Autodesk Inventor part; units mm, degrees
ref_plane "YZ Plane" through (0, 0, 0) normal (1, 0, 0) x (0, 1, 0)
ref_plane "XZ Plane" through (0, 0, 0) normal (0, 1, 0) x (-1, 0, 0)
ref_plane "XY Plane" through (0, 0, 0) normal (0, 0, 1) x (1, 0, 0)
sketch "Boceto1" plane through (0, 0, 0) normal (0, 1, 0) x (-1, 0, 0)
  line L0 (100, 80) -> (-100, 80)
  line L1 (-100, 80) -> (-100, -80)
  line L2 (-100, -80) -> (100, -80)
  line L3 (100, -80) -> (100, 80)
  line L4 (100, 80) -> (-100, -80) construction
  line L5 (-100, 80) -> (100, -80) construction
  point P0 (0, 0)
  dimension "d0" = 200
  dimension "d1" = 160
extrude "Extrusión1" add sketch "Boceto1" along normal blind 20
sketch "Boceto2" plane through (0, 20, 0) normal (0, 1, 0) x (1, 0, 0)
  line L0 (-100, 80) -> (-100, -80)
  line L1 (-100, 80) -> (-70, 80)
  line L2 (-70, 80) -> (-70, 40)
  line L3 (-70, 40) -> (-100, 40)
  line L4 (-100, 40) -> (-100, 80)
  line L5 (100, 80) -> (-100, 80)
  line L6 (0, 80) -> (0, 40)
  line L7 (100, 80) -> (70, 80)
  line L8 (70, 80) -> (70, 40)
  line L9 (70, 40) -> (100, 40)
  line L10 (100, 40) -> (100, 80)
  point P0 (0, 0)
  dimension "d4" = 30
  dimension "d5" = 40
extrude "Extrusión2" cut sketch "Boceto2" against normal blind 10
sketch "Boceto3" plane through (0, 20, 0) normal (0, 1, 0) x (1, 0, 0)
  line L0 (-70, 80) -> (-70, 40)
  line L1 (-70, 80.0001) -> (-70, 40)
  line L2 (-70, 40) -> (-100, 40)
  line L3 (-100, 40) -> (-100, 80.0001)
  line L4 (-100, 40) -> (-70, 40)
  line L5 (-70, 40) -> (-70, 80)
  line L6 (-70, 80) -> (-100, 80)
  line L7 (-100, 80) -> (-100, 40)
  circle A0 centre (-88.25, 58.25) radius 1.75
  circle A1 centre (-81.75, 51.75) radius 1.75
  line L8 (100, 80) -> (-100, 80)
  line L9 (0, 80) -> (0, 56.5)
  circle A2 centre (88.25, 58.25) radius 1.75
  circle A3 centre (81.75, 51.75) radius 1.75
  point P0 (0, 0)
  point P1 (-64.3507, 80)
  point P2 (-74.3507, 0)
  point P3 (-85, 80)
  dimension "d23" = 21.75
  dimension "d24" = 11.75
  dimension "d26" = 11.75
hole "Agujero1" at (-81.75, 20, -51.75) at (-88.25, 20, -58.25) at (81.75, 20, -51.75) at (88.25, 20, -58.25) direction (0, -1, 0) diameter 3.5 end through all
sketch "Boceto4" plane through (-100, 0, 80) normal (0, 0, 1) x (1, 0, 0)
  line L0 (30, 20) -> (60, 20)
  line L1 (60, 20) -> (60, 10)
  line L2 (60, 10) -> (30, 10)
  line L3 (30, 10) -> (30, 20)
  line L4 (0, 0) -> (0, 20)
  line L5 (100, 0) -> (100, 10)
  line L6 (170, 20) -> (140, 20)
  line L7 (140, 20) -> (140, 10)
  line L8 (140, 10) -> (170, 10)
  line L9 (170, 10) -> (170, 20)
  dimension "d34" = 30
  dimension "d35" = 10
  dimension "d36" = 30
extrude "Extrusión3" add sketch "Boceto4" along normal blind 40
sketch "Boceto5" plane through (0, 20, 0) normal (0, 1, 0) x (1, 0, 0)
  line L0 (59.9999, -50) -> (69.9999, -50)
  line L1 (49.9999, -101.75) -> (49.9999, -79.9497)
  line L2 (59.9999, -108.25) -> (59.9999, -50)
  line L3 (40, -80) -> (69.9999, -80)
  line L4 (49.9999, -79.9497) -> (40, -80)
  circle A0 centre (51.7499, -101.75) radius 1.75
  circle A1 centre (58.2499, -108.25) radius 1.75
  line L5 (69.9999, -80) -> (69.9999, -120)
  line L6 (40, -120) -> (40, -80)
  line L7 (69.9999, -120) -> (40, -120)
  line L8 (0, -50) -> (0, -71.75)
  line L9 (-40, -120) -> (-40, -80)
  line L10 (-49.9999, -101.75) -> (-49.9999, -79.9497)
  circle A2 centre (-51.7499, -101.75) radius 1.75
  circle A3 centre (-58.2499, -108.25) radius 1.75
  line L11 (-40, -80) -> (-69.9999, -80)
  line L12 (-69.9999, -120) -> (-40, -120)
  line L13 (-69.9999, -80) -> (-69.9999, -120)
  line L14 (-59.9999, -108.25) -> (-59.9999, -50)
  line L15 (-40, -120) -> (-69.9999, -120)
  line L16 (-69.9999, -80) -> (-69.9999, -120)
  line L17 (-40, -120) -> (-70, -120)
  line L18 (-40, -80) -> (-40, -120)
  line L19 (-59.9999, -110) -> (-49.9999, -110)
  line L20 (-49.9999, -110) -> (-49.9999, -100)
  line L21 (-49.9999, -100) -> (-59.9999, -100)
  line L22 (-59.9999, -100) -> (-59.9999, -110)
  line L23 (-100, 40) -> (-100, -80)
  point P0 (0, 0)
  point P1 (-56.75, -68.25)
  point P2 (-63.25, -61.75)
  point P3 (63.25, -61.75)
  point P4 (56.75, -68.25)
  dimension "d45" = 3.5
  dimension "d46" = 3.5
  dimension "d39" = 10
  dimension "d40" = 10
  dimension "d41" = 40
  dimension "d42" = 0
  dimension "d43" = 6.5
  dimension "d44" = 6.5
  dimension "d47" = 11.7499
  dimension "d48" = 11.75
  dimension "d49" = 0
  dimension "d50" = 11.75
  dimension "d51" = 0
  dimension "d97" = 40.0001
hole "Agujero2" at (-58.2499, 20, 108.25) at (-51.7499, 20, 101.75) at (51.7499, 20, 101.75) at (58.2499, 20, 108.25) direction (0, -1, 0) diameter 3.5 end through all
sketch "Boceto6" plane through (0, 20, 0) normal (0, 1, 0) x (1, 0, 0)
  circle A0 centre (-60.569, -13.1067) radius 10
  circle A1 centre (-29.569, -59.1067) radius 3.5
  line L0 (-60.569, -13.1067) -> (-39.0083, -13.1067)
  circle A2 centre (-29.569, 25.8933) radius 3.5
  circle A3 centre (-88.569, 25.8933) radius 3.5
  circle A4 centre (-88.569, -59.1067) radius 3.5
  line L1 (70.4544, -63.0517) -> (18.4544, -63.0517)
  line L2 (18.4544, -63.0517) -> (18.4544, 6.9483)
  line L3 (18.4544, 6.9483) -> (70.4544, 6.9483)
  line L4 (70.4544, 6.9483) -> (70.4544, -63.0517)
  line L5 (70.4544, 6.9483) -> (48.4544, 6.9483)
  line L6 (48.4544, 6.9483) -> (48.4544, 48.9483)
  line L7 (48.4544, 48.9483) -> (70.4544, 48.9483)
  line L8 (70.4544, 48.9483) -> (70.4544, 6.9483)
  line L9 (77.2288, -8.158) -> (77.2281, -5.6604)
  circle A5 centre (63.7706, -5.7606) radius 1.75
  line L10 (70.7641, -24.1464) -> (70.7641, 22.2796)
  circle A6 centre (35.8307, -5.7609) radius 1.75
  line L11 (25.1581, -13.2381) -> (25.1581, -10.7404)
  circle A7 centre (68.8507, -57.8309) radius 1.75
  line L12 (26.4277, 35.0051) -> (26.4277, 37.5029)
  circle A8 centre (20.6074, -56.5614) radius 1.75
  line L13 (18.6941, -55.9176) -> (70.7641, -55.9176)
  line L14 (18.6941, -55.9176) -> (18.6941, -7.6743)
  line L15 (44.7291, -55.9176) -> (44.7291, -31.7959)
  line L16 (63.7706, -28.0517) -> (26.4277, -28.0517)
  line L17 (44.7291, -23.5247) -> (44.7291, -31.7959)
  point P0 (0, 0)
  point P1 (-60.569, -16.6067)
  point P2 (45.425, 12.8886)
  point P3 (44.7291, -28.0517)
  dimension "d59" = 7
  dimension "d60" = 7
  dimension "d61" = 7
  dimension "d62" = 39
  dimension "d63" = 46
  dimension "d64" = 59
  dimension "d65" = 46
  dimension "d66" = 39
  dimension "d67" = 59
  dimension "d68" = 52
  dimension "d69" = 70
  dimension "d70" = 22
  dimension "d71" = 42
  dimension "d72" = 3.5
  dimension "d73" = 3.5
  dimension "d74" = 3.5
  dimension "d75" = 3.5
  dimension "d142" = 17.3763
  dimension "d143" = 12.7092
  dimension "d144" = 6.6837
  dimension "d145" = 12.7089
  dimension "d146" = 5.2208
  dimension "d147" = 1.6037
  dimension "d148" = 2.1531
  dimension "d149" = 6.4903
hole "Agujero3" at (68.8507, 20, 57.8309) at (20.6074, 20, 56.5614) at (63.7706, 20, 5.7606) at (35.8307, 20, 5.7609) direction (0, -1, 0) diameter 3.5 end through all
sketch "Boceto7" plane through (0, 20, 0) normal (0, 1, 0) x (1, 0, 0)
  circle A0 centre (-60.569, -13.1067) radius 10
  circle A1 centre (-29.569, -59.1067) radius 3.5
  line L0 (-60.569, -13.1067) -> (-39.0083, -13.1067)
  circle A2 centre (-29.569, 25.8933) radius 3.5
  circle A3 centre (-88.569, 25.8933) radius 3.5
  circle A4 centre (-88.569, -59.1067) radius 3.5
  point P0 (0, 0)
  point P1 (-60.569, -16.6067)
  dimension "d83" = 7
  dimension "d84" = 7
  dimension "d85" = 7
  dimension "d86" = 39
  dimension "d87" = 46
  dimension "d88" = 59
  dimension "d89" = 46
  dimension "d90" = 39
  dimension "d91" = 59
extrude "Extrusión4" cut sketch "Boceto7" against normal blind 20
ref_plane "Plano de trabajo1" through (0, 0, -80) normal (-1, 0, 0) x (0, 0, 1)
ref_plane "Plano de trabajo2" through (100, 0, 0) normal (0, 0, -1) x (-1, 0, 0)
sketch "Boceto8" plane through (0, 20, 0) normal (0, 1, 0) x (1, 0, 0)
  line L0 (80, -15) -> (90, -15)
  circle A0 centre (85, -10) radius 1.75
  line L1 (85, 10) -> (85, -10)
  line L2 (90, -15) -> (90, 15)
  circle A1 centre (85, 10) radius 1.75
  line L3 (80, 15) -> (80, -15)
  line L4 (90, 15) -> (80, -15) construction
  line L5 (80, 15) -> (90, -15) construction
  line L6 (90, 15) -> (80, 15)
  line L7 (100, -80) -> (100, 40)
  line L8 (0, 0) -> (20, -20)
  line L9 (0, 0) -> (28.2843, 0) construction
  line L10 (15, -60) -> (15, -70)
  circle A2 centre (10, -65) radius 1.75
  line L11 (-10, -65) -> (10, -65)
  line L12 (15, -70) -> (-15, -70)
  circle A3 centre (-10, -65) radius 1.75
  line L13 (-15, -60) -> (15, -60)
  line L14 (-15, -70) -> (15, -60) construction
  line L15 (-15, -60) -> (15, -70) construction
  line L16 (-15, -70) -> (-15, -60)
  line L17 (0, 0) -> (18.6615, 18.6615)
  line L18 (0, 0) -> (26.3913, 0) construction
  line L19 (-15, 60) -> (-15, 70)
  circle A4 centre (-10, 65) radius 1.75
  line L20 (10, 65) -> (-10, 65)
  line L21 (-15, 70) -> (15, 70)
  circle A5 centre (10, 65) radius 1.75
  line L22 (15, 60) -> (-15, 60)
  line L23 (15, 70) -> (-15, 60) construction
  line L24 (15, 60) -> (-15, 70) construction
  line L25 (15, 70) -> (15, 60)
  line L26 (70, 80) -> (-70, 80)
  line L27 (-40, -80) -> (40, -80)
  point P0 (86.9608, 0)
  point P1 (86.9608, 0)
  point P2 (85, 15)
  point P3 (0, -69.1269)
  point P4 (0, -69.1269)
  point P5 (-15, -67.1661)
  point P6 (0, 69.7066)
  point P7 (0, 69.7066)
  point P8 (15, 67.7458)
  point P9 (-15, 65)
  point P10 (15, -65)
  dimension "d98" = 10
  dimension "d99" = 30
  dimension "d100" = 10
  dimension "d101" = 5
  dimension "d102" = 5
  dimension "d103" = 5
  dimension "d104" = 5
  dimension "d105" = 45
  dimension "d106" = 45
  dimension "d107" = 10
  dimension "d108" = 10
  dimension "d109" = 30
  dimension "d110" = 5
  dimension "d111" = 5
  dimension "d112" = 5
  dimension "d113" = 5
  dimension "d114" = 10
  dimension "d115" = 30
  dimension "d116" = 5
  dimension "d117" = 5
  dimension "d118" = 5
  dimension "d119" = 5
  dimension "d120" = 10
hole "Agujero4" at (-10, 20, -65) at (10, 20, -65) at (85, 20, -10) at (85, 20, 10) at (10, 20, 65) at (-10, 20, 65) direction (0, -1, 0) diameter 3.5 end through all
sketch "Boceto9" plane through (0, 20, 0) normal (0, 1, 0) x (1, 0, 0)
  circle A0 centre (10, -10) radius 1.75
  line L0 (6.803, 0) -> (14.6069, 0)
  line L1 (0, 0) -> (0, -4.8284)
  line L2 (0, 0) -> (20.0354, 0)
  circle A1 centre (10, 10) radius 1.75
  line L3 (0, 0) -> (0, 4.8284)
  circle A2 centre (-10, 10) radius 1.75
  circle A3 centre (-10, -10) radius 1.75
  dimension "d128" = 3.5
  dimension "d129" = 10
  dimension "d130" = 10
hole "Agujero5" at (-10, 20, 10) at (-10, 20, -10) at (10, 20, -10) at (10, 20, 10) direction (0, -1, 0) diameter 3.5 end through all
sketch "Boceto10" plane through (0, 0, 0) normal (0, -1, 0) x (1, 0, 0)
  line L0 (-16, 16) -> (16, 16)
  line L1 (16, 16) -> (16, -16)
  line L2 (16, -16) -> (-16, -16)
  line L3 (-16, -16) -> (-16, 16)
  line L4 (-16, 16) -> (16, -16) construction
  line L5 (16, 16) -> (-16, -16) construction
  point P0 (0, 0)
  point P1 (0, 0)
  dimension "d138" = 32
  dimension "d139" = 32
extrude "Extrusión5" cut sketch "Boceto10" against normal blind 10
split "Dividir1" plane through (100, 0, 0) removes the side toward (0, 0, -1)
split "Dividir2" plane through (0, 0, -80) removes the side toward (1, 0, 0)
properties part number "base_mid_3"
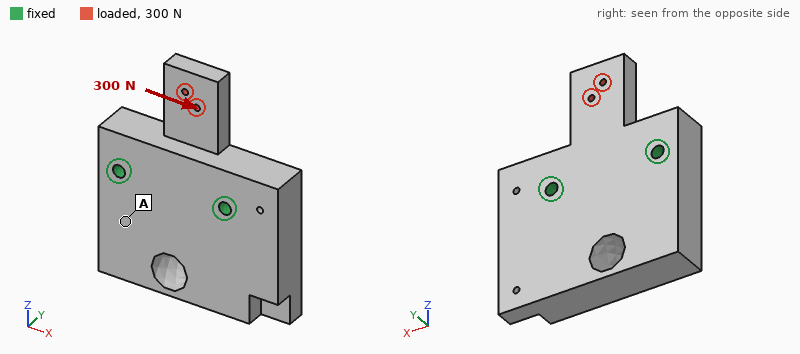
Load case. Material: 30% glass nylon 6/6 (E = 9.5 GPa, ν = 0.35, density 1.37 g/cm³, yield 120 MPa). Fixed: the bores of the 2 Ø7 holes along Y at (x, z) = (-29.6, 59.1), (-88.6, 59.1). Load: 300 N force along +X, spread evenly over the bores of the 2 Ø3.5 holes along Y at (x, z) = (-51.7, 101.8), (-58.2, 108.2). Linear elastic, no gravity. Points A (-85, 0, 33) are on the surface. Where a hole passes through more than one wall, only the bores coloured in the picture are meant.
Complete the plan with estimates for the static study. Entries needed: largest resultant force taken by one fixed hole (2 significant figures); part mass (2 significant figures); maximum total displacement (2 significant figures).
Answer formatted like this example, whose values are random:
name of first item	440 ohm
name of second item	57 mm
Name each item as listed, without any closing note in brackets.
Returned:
largest resultant force taken by one fixed hole	280 N
part mass	220 g
maximum total displacement	39 µm
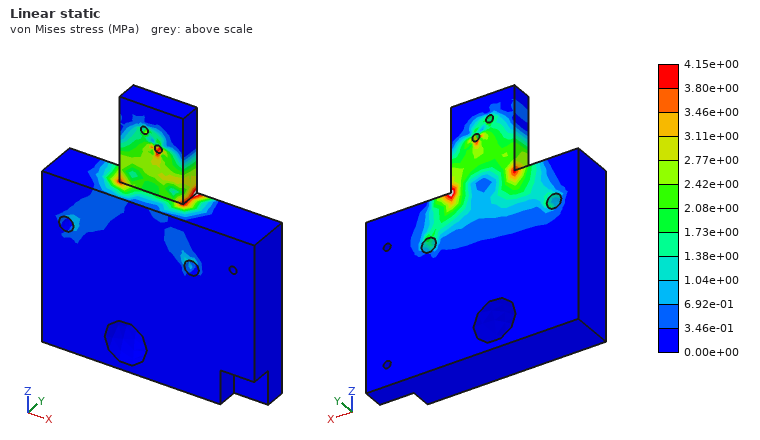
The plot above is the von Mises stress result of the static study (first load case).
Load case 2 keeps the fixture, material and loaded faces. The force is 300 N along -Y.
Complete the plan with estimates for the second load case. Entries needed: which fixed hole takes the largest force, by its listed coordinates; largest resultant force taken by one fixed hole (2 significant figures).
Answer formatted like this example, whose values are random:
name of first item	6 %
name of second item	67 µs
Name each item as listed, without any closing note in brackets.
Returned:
which fixed hole takes the largest force, by its listed coordinates	(-29.6, 59.1)
largest resultant force taken by one fixed hole	180 N
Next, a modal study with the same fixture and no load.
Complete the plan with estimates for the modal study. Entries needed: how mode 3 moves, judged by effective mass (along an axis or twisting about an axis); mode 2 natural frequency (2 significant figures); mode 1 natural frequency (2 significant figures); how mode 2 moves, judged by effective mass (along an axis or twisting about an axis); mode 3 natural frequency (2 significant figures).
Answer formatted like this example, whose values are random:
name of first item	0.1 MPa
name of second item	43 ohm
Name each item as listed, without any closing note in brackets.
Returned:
how mode 3 moves, judged by effective mass	twisting about Z
mode 2 natural frequency	2100 Hz
mode 1 natural frequency	1800 Hz
how mode 2 moves, judged by effective mass	along Y
mode 3 natural frequency	3100 Hz
